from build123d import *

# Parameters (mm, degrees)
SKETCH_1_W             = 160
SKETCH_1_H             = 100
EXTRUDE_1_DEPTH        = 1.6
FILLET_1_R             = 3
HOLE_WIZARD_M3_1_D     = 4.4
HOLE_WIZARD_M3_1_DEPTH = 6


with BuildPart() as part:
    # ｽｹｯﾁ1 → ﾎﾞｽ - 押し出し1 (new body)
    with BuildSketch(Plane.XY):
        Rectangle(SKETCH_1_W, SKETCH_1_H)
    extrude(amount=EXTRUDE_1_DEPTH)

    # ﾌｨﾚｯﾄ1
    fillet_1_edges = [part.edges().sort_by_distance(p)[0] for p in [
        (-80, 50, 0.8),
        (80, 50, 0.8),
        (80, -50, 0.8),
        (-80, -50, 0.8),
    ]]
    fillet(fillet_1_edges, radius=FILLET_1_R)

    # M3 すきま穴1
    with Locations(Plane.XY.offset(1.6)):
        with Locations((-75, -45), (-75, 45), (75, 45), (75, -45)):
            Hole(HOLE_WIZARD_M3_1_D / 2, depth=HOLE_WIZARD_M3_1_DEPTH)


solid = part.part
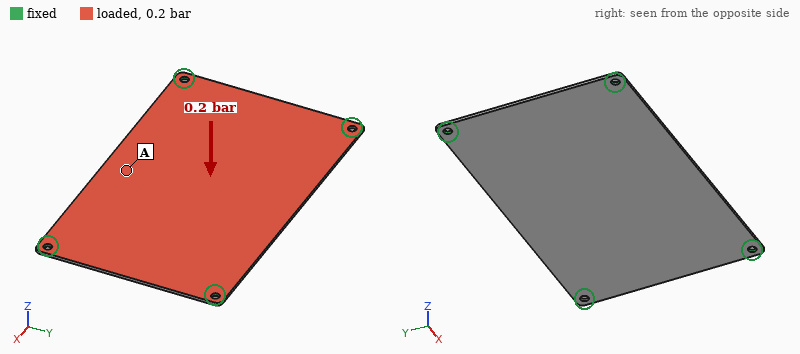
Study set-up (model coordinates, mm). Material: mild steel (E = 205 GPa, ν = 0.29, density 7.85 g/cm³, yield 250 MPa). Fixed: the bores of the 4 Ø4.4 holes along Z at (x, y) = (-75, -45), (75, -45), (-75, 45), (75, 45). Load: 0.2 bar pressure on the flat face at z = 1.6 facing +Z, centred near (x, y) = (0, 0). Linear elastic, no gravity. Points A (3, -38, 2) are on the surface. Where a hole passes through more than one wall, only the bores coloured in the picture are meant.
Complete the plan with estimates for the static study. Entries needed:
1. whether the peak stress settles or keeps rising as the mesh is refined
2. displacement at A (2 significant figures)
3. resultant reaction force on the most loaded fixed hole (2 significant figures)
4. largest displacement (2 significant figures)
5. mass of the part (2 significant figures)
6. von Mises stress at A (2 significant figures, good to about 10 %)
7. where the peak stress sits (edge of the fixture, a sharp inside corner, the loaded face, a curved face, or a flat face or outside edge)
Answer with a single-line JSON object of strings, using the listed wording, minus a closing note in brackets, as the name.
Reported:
{"whether the peak stress settles or keeps rising as the mesh is refined": "keeps rising", "displacement at A": "0.57 mm", "resultant reaction force on the most loaded fixed hole": "80 N", "largest displacement": "0.59 mm", "mass of the part": "200 g", "von Mises stress at A": "55 MPa", "where the peak stress sits": "edge of the fixture"}
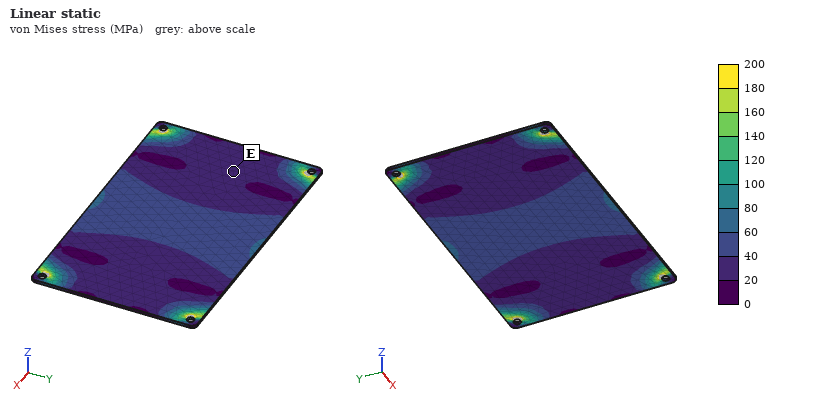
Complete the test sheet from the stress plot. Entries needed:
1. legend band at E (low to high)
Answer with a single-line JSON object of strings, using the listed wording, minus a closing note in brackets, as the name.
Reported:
{"legend band at E": "20 to 40 MPa"}
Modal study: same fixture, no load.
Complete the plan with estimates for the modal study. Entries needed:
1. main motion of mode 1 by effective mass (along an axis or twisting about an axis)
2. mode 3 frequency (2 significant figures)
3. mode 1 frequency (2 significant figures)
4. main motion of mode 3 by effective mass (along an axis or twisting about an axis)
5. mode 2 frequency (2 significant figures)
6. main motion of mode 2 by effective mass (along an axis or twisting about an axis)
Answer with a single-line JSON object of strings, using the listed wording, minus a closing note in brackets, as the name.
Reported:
{"main motion of mode 1 by effective mass": "along Z", "mode 3 frequency": "780 Hz", "mode 1 frequency": "300 Hz", "main motion of mode 3 by effective mass": "twisting about Y", "mode 2 frequency": "530 Hz", "main motion of mode 2 by effective mass": "twisting about X"}
